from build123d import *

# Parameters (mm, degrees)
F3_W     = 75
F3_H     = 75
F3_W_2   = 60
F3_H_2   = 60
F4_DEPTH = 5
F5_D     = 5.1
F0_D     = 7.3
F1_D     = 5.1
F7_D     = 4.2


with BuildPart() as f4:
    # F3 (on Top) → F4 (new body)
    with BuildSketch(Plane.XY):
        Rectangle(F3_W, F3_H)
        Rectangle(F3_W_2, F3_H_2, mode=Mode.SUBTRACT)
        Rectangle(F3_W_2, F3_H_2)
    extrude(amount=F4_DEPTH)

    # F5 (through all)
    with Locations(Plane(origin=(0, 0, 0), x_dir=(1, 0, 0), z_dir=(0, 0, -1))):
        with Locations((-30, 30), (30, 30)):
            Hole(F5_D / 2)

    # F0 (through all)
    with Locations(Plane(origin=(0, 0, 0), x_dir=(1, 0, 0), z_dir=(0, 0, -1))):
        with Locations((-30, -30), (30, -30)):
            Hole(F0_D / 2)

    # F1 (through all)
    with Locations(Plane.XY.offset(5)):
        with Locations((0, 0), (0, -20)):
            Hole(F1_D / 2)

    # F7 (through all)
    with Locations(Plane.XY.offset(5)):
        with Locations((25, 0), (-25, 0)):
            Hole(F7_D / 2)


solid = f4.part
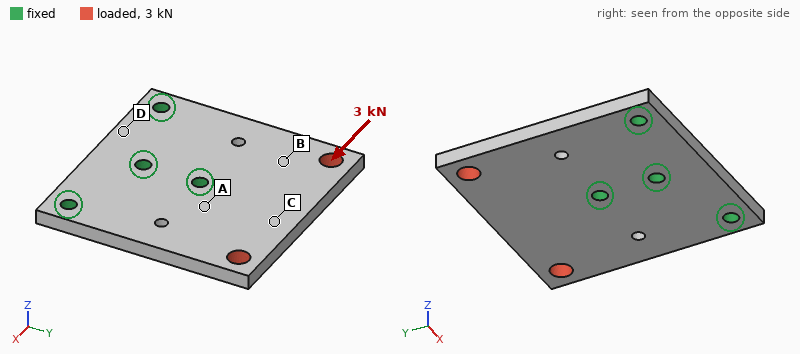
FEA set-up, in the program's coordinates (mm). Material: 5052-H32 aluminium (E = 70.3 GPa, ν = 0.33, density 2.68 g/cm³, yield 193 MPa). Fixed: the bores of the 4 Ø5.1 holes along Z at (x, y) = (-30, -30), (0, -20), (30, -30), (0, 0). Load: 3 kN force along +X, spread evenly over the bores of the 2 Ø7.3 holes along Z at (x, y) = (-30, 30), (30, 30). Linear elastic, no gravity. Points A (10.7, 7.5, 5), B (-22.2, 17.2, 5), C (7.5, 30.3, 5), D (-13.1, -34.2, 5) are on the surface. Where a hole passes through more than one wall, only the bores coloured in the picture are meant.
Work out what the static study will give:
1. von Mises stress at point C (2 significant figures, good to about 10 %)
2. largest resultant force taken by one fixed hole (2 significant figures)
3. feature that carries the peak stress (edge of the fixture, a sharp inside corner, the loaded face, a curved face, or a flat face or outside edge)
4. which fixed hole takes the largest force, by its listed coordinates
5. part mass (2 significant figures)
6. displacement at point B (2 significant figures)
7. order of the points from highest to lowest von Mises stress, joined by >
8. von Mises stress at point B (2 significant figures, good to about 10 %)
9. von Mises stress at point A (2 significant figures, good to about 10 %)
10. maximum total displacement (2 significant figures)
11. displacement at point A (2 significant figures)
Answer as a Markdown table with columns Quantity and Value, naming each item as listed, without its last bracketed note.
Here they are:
| Quantity | Value |
|---|---|
| von Mises stress at point C | 10 MPa |
| largest resultant force taken by one fixed hole | 3.1 kN |
| feature that carries the peak stress | edge of the fixture |
| which fixed hole takes the largest force, by its listed coordinates | (0, 0) |
| part mass | 73 g |
| displacement at point B | 16 µm |
| order of the points from highest to lowest von Mises stress, joined by > | A > B > C > D |
| von Mises stress at point B | 17 MPa |
| von Mises stress at point A | 22 MPa |
| maximum total displacement | 33 µm |
| displacement at point A | 7.6 µm |
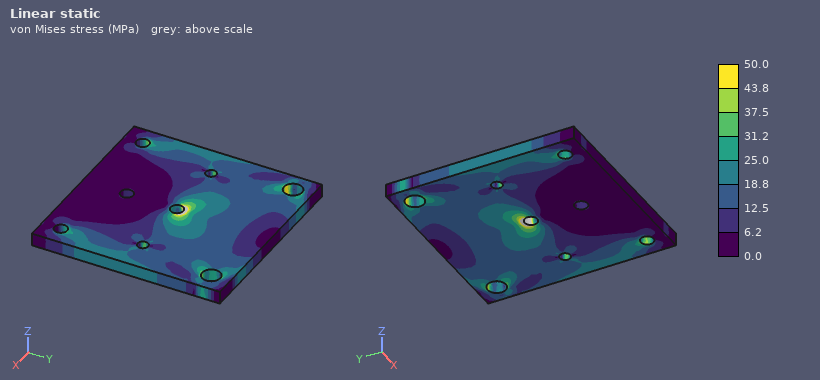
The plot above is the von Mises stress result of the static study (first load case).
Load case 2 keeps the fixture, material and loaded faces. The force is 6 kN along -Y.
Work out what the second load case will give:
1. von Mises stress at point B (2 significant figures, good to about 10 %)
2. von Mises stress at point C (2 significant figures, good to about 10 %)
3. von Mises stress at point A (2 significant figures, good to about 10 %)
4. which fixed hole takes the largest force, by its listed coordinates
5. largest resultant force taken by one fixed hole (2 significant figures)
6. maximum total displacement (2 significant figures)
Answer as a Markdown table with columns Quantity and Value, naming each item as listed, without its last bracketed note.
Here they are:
| Quantity | Value |
|---|---|
| von Mises stress at point B | 22 MPa |
| von Mises stress at point C | 13 MPa |
| von Mises stress at point A | 15 MPa |
| which fixed hole takes the largest force, by its listed coordinates | (0, 0) |
| largest resultant force taken by one fixed hole | 2.1 kN |
| maximum total displacement | 27 µm |
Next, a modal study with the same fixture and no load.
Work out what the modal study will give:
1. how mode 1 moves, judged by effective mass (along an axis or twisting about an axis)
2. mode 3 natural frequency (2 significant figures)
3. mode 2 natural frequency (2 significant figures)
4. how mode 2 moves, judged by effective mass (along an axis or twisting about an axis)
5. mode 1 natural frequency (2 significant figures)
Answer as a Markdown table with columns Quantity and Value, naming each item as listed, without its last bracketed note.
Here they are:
| Quantity | Value |
|---|---|
| how mode 1 moves, judged by effective mass | along Z |
| mode 3 natural frequency | 5600 Hz |
| mode 2 natural frequency | 2500 Hz |
| how mode 2 moves, judged by effective mass | twisting about Y |
| mode 1 natural frequency | 2300 Hz |
